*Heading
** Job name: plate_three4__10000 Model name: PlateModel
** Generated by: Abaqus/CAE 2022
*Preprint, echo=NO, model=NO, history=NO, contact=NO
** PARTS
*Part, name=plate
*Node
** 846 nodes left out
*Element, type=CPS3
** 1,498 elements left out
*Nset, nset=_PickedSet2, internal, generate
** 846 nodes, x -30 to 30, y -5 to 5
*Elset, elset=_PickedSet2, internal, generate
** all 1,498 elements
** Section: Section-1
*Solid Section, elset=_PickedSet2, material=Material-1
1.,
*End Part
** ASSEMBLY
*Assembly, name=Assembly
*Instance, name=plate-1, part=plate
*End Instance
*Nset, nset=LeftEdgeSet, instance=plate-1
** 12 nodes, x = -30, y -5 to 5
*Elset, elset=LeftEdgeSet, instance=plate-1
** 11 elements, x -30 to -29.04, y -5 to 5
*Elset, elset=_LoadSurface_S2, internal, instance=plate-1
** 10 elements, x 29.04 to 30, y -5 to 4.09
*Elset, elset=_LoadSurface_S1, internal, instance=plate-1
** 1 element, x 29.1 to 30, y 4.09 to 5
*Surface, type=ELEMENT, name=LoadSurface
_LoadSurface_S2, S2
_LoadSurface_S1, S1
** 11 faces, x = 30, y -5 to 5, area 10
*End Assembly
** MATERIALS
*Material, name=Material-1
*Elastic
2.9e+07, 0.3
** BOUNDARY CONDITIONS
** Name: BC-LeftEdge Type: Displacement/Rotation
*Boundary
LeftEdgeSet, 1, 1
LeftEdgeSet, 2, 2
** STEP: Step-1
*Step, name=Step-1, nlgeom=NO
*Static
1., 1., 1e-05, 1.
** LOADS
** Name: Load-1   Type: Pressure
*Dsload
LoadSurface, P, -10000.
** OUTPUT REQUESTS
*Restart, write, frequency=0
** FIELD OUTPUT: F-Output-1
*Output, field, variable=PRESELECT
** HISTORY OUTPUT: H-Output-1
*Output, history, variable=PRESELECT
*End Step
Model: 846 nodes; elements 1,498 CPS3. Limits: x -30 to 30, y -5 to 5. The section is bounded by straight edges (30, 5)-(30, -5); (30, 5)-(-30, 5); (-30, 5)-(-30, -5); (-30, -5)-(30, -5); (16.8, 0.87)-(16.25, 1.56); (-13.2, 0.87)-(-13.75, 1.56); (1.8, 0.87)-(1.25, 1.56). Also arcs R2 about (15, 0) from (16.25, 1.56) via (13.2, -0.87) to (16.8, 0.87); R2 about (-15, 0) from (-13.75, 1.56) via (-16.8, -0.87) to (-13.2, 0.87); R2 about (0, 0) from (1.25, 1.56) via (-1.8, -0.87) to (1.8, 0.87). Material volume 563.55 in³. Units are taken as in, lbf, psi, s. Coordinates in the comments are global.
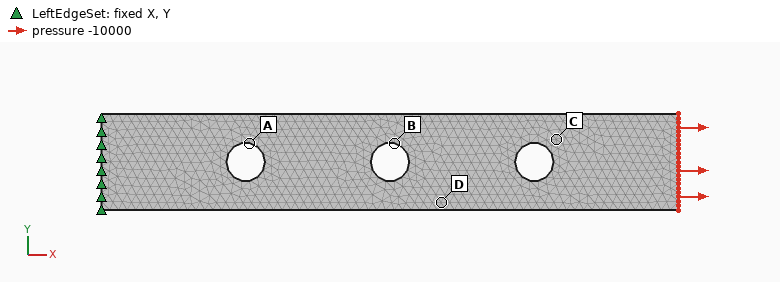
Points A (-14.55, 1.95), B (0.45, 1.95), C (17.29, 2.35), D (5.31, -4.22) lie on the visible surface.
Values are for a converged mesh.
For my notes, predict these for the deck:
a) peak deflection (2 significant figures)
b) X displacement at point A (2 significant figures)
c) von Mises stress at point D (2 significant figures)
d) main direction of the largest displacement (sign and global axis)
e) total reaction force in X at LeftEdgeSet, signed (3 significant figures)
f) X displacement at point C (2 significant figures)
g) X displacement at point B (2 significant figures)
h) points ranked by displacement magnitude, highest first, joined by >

0.025 in
0.0064 in
13000 psi
+X
-1.00e+05 lbf
0.021 in
0.013 in
C > D > B > A
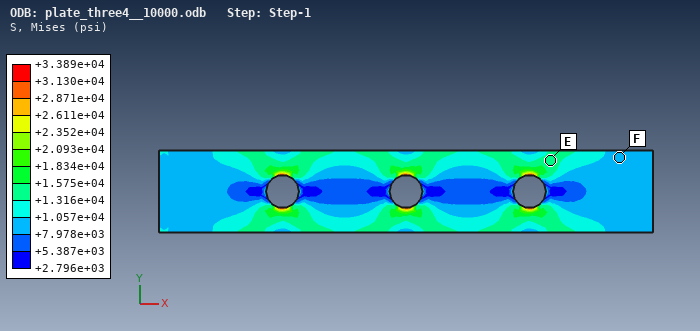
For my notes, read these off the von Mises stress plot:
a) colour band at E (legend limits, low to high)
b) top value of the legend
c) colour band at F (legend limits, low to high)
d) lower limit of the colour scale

+1.316e+04 to +1.575e+04 psi
+3.389e+04 psi
+7.978e+03 to +1.057e+04 psi
+2.796e+03 psi
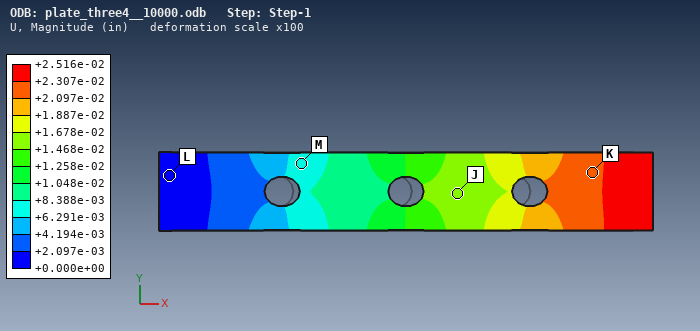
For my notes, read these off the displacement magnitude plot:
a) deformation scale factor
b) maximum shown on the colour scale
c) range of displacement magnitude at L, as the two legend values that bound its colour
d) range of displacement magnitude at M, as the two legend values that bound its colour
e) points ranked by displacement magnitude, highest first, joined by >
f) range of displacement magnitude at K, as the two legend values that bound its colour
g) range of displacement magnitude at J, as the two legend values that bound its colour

100
+2.516e-02 in
+0.000e+00 to +2.097e-03 in
+6.291e-03 to +8.388e-03 in
K > J > M > L
+2.097e-02 to +2.307e-02 in
+1.468e-02 to +1.678e-02 in
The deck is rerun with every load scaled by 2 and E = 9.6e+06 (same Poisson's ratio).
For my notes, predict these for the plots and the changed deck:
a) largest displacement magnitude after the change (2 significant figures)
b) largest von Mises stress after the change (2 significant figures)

0.15 in
68000 psi
